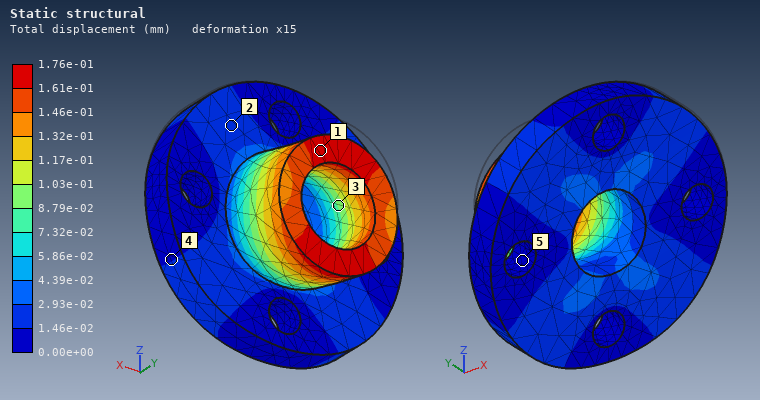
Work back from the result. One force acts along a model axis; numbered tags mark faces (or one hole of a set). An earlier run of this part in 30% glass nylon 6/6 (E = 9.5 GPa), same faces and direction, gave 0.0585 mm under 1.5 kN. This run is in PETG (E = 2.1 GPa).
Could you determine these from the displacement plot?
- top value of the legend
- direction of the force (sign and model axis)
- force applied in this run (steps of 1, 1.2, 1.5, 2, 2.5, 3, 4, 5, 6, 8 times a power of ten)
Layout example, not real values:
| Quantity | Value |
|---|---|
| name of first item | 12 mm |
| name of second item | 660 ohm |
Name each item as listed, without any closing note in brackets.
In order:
| Quantity | Value |
|---|---|
| top value of the legend | 1.76e-01 mm |
| direction of the force | -Z |
| force applied in this run | 1 kN |
